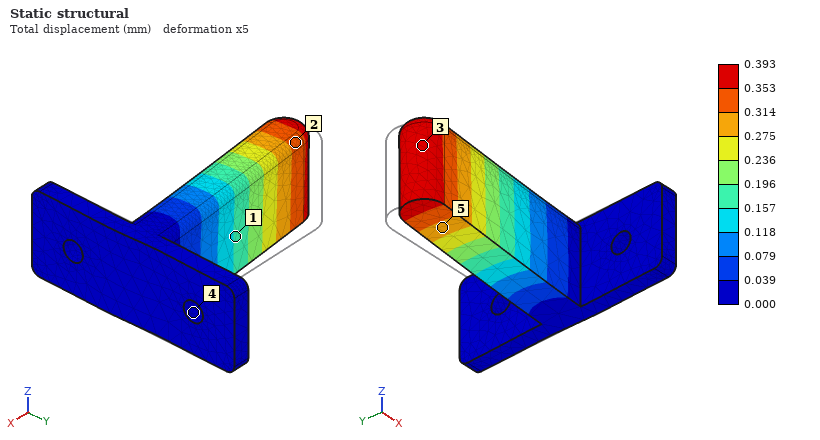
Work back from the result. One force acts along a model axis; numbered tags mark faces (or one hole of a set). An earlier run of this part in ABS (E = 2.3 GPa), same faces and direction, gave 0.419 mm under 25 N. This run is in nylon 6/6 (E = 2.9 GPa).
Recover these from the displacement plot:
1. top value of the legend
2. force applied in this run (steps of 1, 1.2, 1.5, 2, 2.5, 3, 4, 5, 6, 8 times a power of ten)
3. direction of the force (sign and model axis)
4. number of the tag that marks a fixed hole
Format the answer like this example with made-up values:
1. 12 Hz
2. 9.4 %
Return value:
1. 0.393 mm
2. 30 N
3. -Y
4. 4
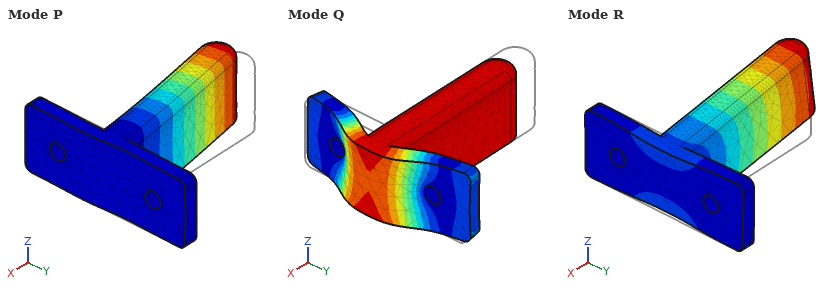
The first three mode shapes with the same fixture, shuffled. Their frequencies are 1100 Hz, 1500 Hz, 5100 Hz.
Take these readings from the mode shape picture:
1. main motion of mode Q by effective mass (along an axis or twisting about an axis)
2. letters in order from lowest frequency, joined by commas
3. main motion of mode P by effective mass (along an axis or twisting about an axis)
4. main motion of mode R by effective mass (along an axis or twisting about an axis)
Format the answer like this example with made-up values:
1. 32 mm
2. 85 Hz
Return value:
1. along X
2. R, P, Q
3. along Y
4. along Z
